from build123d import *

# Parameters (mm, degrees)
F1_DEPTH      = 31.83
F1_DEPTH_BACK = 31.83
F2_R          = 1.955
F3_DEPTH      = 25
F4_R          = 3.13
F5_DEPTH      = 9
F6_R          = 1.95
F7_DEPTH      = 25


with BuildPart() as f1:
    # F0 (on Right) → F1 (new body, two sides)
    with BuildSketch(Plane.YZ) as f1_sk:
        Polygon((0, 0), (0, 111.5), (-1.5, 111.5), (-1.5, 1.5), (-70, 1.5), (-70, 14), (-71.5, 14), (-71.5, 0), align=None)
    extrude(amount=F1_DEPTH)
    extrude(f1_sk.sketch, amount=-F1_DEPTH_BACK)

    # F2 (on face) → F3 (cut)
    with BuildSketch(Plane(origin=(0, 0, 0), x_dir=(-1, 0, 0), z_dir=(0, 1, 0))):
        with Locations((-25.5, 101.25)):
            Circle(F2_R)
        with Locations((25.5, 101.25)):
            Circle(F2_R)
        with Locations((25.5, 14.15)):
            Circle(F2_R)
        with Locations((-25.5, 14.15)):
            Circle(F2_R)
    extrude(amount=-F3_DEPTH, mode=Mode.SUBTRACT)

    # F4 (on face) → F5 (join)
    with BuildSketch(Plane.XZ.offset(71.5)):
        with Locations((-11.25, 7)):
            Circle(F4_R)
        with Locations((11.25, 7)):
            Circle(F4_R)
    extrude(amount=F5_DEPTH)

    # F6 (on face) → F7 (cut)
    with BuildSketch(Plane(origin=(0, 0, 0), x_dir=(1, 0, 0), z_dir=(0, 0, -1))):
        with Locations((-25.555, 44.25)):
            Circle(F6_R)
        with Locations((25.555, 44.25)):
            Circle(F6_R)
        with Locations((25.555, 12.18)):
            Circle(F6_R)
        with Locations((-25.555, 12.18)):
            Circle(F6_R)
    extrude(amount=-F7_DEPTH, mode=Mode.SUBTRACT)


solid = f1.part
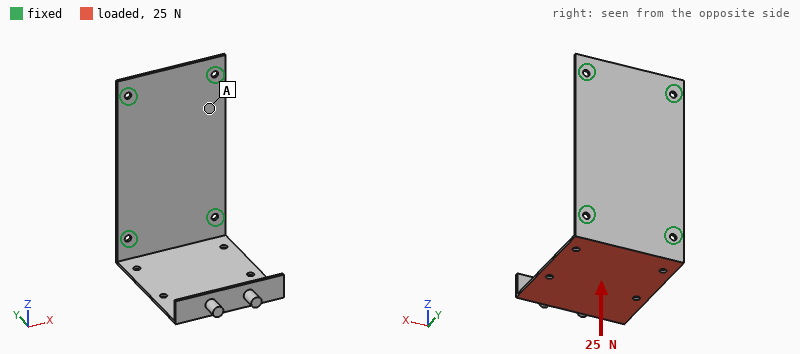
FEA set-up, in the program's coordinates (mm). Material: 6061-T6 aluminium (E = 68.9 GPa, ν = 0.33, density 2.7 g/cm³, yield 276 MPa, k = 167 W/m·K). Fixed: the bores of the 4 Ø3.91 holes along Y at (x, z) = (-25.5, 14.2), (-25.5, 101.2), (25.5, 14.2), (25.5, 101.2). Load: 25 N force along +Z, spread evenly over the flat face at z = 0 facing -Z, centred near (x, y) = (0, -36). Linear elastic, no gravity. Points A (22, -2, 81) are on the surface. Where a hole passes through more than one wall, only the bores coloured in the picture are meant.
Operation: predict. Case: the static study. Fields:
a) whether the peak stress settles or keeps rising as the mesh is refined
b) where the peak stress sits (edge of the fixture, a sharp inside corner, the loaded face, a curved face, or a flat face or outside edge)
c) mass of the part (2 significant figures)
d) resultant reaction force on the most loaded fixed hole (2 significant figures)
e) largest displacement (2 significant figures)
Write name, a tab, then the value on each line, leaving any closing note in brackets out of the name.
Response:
whether the peak stress settles or keeps rising as the mesh is refined	keeps rising
where the peak stress sits	edge of the fixture
mass of the part	51 g
resultant reaction force on the most loaded fixed hole	9.7 N
largest displacement	1.7 mm
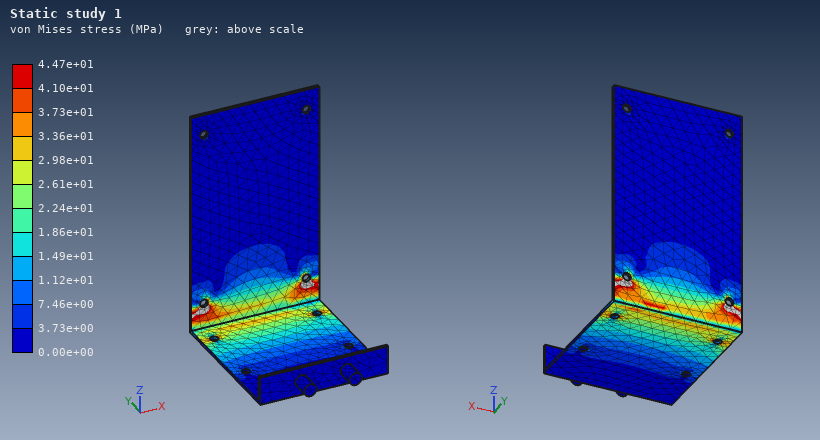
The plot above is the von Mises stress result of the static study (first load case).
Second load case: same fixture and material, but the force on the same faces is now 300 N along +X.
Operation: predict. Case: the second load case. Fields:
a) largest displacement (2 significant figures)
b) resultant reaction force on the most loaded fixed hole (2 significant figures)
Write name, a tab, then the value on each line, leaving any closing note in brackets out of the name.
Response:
largest displacement	0.92 mm
resultant reaction force on the most loaded fixed hole	270 N
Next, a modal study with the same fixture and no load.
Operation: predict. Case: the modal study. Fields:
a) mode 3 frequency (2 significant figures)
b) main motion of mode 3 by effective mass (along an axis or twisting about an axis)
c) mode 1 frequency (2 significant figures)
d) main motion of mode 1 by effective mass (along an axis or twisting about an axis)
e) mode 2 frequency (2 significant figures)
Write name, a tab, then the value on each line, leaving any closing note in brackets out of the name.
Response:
mode 3 frequency	780 Hz
main motion of mode 3 by effective mass	along X
mode 1 frequency	130 Hz
main motion of mode 1 by effective mass	along Z
mode 2 frequency	440 Hz
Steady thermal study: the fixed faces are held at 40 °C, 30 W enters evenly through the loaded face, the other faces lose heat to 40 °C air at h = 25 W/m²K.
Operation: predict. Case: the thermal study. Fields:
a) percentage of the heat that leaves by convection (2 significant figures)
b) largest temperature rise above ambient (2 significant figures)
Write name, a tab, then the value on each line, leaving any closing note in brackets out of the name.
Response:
percentage of the heat that leaves by convection	37 %
largest temperature rise above ambient	63 K
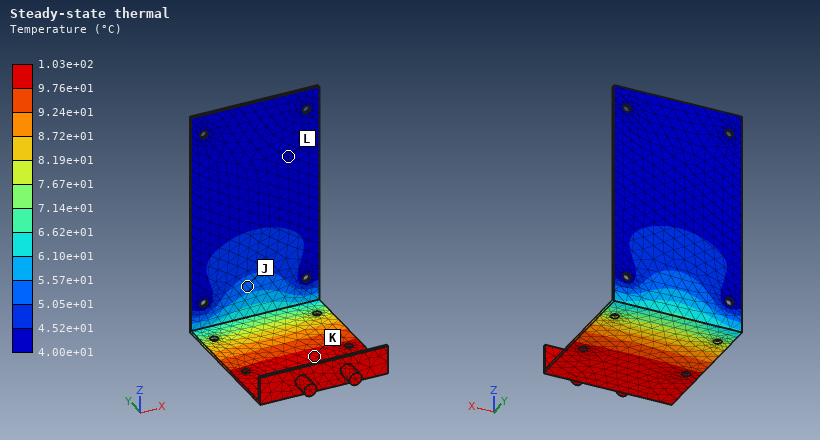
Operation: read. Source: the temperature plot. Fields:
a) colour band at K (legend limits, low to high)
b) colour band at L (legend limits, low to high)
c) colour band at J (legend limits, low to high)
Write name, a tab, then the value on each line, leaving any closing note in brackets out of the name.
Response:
colour band at K	9.76e+01 to 1.03e+02 °C
colour band at L	4.00e+01 to 4.52e+01 °C
colour band at J	5.05e+01 to 5.57e+01 °C
